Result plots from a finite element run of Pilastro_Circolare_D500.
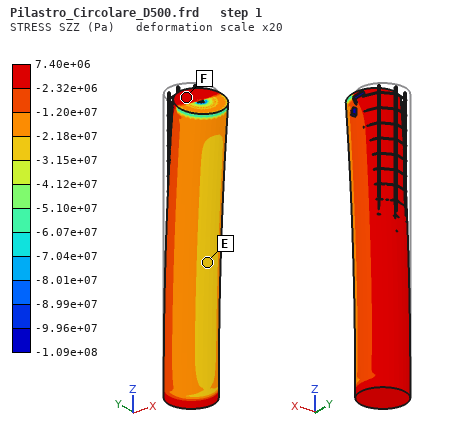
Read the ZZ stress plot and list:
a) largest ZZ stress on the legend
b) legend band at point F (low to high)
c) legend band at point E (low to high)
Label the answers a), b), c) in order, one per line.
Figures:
a) 7.40e+06 Pa
b) -2.32e+06 to 7.40e+06 Pa
c) -3.15e+07 to -2.18e+07 Pa
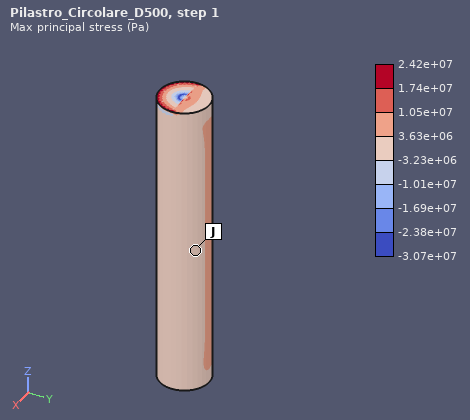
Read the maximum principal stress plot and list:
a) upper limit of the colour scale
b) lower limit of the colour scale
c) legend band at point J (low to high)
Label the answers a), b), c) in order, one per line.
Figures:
a) 2.42e+07 Pa
b) -3.07e+07 Pa
c) -3.23e+06 to 3.63e+06 Pa
